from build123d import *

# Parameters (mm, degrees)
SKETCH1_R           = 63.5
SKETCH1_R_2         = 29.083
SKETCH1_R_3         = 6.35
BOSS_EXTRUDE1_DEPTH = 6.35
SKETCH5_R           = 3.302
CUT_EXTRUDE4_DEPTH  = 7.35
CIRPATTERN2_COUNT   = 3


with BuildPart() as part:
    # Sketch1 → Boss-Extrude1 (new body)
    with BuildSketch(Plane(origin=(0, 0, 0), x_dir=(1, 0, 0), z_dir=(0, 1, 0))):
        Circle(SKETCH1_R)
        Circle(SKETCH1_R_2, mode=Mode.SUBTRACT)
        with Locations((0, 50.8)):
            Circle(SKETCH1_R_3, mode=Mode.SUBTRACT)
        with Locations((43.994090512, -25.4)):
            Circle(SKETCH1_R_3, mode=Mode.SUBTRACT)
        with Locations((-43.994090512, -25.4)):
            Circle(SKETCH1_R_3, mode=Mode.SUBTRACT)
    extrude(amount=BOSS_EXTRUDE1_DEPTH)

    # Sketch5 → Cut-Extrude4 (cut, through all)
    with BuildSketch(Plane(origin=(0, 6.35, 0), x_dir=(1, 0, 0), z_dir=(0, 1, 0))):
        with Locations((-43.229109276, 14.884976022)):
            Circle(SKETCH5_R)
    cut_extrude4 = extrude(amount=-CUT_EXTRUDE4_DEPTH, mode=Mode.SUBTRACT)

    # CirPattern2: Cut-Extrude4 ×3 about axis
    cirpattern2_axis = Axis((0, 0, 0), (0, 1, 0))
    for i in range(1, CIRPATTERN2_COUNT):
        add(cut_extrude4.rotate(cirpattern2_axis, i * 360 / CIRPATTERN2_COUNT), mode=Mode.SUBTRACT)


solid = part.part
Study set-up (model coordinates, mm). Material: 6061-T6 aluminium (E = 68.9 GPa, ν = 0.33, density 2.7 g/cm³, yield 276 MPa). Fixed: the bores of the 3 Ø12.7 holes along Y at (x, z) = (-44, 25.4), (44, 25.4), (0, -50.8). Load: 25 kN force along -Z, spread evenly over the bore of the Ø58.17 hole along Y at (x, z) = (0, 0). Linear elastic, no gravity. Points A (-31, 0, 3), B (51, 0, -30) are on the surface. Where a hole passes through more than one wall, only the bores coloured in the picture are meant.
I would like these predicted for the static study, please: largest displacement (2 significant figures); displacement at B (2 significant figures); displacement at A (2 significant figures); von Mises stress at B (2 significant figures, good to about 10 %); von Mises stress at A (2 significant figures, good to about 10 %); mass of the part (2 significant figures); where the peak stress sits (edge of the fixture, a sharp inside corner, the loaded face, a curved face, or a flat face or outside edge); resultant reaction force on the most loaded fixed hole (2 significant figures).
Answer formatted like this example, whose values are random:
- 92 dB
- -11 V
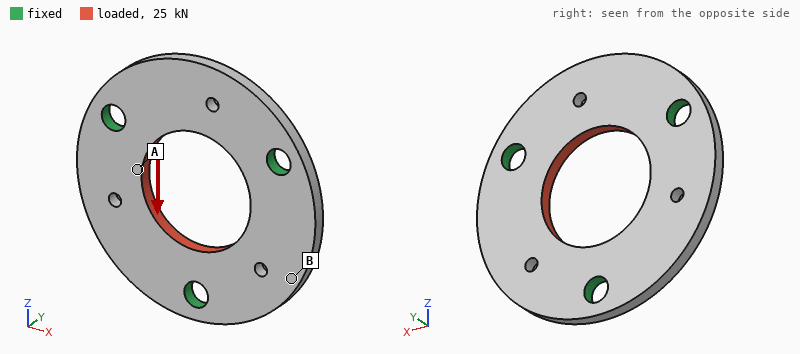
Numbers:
- 35 µm
- 15 µm
- 18 µm
- 15 MPa
- 36 MPa
- 160 g
- edge of the fixture
- 9.2 kN
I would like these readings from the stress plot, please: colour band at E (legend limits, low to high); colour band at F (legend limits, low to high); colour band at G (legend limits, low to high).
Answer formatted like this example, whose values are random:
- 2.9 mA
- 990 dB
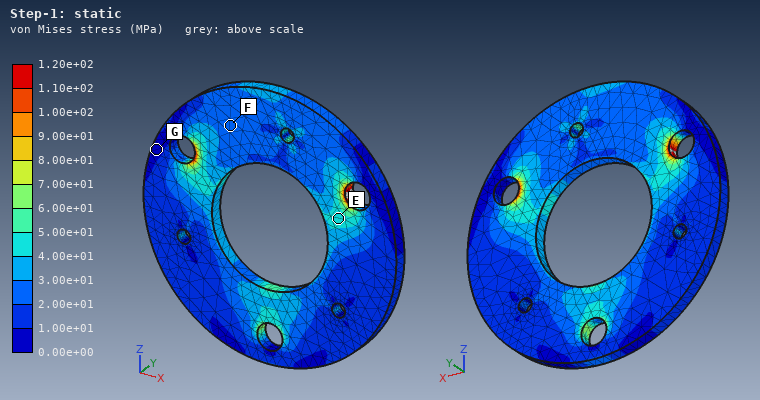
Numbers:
- 4.00e+01 to 5.00e+01 MPa
- 2.00e+01 to 3.00e+01 MPa
- 0.00e+00 to 1.00e+01 MPa
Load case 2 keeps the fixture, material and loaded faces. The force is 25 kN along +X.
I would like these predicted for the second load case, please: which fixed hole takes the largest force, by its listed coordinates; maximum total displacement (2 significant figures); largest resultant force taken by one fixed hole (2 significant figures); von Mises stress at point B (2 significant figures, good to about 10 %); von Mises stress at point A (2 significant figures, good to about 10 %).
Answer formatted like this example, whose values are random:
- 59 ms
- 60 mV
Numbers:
- (0, -50.8)
- 31 µm
- 9.9 kN
- 26 MPa
- 25 MPa
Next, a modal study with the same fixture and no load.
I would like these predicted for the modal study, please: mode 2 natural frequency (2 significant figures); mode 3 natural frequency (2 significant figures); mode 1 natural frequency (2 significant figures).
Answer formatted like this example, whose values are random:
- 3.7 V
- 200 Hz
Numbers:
- 3100 Hz
- 3200 Hz
- 3100 Hz
